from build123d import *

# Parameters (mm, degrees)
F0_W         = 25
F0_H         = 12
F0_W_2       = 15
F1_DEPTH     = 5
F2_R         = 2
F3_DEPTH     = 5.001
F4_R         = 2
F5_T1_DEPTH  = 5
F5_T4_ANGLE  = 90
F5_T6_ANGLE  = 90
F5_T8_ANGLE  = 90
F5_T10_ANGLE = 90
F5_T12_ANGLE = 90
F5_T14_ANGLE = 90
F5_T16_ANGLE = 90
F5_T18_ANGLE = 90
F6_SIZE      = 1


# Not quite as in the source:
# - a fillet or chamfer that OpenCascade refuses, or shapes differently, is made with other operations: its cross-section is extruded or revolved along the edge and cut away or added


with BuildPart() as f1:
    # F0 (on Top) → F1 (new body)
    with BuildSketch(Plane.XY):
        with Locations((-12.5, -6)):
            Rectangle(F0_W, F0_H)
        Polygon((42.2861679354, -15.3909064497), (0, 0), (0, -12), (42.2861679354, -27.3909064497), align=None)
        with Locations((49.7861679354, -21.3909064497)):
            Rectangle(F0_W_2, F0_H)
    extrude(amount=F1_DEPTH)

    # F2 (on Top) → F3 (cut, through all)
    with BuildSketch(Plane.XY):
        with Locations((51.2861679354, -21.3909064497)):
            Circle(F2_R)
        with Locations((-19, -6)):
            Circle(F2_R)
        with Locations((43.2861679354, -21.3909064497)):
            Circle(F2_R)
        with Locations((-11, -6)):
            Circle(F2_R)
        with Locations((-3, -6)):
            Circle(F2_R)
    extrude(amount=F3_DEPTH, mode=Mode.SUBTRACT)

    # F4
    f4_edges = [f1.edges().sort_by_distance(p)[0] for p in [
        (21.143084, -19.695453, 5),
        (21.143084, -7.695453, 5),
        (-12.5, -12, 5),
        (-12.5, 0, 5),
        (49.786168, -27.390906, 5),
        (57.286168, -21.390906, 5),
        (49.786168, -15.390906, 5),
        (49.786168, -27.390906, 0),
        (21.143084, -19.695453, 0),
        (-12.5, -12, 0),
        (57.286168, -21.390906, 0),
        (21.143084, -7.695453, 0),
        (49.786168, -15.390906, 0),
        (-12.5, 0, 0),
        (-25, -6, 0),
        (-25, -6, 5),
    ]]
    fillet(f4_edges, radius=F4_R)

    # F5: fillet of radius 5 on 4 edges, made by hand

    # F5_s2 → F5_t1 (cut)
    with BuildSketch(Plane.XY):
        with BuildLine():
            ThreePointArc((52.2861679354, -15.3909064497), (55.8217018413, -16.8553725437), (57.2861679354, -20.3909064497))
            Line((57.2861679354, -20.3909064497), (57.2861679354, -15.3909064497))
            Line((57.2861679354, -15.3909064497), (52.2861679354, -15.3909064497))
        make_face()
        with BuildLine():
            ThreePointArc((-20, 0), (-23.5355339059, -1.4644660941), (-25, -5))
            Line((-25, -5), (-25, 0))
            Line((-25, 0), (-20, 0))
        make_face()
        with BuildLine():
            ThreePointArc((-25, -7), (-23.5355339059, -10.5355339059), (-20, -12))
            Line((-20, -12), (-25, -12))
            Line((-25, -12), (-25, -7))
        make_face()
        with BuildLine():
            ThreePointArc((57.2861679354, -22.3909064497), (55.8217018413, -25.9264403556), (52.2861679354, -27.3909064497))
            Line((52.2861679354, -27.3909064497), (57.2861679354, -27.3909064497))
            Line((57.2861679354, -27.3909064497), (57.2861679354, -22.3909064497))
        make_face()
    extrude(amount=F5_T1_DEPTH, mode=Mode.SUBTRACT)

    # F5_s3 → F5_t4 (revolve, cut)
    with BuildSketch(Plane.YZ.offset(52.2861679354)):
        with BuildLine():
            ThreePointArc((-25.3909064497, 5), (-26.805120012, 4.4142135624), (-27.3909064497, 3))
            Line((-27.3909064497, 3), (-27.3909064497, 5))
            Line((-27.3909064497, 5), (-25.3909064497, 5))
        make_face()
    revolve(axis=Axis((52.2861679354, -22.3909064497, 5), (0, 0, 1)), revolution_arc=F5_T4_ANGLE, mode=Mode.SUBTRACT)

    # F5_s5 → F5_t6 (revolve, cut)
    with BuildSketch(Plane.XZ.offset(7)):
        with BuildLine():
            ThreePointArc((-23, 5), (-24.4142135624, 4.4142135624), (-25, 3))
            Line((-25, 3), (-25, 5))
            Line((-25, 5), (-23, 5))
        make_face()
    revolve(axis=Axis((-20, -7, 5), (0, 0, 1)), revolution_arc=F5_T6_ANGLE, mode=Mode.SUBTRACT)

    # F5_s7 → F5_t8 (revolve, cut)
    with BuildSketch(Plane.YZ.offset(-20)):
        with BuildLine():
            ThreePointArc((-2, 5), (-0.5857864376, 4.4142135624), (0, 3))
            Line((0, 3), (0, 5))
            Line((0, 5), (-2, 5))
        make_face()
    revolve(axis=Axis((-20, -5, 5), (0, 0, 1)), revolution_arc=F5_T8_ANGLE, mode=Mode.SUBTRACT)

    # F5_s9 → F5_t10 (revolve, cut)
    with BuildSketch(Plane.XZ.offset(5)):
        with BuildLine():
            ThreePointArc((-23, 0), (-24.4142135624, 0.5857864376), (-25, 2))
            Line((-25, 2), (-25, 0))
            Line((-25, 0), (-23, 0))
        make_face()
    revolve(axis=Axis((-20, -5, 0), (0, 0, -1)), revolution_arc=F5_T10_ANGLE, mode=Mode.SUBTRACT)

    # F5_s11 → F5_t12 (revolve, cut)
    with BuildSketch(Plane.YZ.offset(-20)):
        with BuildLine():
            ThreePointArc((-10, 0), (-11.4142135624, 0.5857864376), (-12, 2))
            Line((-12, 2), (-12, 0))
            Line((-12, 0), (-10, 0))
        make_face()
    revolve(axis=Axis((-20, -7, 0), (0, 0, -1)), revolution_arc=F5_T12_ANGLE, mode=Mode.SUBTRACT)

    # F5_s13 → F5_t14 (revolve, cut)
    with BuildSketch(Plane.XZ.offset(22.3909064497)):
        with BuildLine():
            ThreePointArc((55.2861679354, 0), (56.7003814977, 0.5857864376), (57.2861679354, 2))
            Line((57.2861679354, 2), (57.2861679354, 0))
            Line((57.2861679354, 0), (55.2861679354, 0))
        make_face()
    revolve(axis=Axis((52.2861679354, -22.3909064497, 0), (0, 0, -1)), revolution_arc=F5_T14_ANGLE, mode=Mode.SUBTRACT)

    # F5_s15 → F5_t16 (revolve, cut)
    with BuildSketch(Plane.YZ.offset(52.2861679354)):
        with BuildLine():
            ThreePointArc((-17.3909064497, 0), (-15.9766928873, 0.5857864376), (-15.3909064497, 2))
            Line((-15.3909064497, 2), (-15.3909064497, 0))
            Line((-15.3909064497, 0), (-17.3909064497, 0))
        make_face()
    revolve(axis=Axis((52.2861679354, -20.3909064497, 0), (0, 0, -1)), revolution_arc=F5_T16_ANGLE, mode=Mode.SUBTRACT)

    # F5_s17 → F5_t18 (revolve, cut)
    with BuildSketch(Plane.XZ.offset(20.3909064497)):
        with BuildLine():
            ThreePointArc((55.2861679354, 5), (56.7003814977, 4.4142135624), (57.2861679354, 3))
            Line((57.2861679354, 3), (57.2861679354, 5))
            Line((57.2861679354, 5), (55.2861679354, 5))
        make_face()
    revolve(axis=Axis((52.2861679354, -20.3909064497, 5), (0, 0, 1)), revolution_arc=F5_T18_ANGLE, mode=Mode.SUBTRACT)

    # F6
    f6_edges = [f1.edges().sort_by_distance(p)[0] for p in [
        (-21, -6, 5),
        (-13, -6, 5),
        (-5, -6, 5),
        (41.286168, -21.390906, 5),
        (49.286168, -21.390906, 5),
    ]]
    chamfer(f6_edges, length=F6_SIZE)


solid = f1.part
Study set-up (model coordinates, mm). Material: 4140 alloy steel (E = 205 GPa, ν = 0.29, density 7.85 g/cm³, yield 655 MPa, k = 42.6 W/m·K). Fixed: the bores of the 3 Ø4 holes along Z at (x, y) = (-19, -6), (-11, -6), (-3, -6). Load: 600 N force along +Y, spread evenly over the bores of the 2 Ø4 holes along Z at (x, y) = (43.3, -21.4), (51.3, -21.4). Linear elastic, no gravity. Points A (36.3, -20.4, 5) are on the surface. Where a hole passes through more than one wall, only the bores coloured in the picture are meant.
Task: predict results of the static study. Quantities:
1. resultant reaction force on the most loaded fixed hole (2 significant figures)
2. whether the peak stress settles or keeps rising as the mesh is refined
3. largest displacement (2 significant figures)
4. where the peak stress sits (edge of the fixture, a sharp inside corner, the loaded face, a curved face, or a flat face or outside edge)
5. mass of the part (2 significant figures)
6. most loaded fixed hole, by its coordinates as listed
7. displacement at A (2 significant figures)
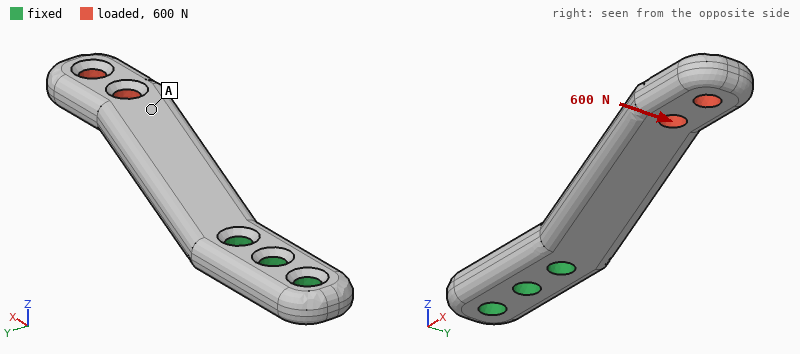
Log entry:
2.0 kN
keeps rising
0.39 mm
edge of the fixture
33 g
(-3, -6)
0.21 mm
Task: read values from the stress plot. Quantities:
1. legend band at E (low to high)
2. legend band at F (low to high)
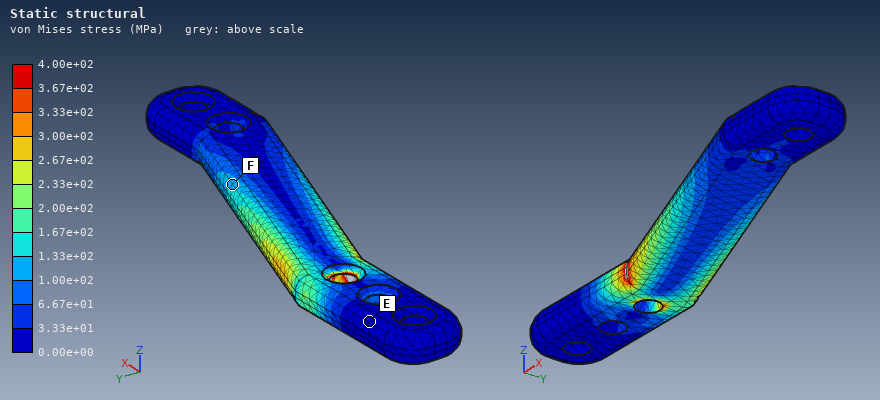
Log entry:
0.00e+00 to 3.33e+01 MPa
1.00e+02 to 1.33e+02 MPa
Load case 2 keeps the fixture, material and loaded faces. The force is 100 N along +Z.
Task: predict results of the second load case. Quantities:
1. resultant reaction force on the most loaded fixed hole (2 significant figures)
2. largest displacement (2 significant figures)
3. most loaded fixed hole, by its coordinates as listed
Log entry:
240 N
0.29 mm
(-3, -6)
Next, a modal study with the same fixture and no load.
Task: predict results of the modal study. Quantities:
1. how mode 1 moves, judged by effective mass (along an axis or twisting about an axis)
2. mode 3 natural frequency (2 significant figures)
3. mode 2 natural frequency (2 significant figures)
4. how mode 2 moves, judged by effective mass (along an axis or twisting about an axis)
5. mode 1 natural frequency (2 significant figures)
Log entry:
along Z
6300 Hz
2200 Hz
along Y
1100 Hz
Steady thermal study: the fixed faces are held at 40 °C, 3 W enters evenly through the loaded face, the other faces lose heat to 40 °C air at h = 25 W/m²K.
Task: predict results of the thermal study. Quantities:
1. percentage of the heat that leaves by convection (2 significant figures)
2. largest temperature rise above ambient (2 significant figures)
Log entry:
40 %
51 K
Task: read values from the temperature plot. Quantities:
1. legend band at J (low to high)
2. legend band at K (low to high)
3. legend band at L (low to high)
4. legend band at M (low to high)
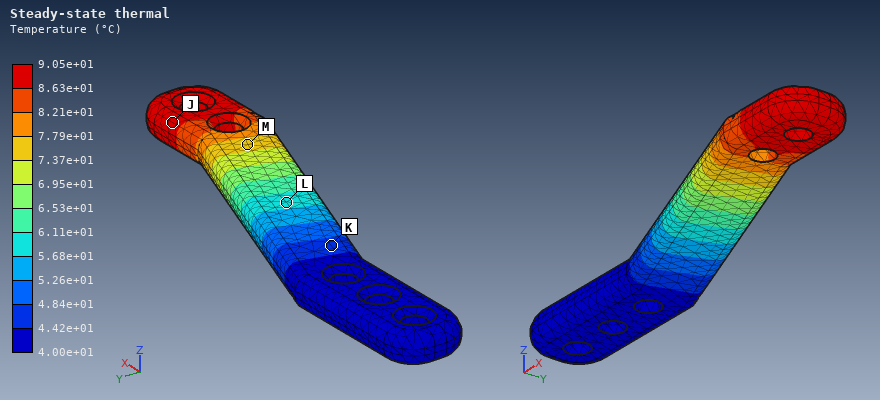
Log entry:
8.63e+01 to 9.05e+01 °C
4.42e+01 to 4.84e+01 °C
5.68e+01 to 6.11e+01 °C
7.37e+01 to 7.79e+01 °C
